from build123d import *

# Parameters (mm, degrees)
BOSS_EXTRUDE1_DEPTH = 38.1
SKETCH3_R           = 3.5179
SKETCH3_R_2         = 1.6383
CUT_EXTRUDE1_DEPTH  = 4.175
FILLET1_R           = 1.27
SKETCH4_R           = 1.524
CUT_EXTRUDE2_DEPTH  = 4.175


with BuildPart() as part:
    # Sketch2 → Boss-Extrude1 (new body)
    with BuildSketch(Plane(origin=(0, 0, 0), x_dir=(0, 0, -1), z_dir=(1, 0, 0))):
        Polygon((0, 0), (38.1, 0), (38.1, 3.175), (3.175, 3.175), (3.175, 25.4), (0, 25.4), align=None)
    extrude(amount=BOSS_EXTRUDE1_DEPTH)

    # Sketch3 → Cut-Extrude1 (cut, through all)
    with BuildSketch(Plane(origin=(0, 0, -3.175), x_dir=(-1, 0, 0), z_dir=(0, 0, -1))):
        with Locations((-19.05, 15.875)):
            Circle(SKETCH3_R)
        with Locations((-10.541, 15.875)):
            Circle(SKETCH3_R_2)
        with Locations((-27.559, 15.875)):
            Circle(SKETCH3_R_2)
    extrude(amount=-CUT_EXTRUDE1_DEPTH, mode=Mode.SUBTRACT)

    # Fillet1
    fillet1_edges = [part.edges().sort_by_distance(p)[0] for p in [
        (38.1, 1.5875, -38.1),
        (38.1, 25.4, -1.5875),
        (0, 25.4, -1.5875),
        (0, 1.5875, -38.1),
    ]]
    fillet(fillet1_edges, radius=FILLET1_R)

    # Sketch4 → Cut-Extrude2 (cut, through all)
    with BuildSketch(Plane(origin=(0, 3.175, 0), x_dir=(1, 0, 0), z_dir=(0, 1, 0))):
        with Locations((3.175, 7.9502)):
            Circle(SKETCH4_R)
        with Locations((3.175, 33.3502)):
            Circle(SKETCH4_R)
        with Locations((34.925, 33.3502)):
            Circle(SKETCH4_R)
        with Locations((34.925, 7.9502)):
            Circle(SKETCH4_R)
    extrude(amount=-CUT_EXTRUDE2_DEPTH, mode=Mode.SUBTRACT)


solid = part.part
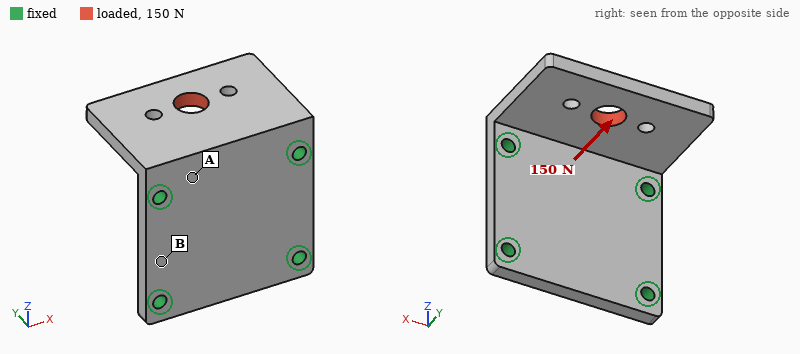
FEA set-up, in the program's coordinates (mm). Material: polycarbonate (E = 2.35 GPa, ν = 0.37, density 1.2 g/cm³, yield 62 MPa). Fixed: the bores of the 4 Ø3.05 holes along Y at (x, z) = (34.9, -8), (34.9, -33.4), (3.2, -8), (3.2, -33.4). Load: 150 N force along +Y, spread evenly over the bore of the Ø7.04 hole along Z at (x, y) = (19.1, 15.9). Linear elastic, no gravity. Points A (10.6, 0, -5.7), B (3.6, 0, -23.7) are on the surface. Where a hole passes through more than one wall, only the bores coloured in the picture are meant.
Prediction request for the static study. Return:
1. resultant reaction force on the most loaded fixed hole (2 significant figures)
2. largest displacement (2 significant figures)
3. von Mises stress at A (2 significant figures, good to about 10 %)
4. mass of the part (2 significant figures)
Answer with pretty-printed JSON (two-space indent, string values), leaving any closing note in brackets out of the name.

{
  "resultant reaction force on the most loaded fixed hole": "82 N",
  "largest displacement": "0.38 mm",
  "von Mises stress at A": "4.6 MPa",
  "mass of the part": "8.4 g"
}
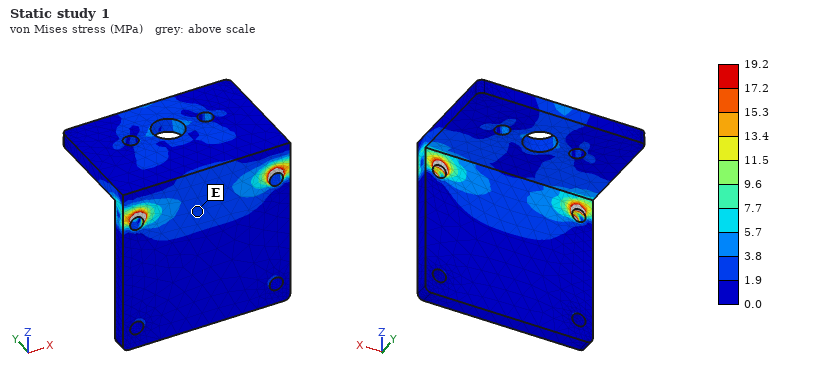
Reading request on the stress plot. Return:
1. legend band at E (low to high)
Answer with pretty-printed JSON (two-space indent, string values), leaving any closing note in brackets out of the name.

{
  "legend band at E": "1.9 to 3.8 MPa"
}
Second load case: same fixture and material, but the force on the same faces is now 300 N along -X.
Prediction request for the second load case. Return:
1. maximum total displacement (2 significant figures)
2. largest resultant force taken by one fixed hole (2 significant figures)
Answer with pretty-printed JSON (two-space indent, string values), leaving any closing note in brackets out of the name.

{
  "maximum total displacement": "0.43 mm",
  "largest resultant force taken by one fixed hole": "210 N"
}
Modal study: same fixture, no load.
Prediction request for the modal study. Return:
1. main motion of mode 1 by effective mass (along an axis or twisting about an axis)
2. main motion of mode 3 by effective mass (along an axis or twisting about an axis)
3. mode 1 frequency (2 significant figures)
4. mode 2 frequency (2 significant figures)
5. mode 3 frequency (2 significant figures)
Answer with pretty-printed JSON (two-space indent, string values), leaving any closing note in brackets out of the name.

{
  "main motion of mode 1 by effective mass": "along Z",
  "main motion of mode 3 by effective mass": "along X",
  "mode 1 frequency": "920 Hz",
  "mode 2 frequency": "1800 Hz",
  "mode 3 frequency": "3500 Hz"
}
